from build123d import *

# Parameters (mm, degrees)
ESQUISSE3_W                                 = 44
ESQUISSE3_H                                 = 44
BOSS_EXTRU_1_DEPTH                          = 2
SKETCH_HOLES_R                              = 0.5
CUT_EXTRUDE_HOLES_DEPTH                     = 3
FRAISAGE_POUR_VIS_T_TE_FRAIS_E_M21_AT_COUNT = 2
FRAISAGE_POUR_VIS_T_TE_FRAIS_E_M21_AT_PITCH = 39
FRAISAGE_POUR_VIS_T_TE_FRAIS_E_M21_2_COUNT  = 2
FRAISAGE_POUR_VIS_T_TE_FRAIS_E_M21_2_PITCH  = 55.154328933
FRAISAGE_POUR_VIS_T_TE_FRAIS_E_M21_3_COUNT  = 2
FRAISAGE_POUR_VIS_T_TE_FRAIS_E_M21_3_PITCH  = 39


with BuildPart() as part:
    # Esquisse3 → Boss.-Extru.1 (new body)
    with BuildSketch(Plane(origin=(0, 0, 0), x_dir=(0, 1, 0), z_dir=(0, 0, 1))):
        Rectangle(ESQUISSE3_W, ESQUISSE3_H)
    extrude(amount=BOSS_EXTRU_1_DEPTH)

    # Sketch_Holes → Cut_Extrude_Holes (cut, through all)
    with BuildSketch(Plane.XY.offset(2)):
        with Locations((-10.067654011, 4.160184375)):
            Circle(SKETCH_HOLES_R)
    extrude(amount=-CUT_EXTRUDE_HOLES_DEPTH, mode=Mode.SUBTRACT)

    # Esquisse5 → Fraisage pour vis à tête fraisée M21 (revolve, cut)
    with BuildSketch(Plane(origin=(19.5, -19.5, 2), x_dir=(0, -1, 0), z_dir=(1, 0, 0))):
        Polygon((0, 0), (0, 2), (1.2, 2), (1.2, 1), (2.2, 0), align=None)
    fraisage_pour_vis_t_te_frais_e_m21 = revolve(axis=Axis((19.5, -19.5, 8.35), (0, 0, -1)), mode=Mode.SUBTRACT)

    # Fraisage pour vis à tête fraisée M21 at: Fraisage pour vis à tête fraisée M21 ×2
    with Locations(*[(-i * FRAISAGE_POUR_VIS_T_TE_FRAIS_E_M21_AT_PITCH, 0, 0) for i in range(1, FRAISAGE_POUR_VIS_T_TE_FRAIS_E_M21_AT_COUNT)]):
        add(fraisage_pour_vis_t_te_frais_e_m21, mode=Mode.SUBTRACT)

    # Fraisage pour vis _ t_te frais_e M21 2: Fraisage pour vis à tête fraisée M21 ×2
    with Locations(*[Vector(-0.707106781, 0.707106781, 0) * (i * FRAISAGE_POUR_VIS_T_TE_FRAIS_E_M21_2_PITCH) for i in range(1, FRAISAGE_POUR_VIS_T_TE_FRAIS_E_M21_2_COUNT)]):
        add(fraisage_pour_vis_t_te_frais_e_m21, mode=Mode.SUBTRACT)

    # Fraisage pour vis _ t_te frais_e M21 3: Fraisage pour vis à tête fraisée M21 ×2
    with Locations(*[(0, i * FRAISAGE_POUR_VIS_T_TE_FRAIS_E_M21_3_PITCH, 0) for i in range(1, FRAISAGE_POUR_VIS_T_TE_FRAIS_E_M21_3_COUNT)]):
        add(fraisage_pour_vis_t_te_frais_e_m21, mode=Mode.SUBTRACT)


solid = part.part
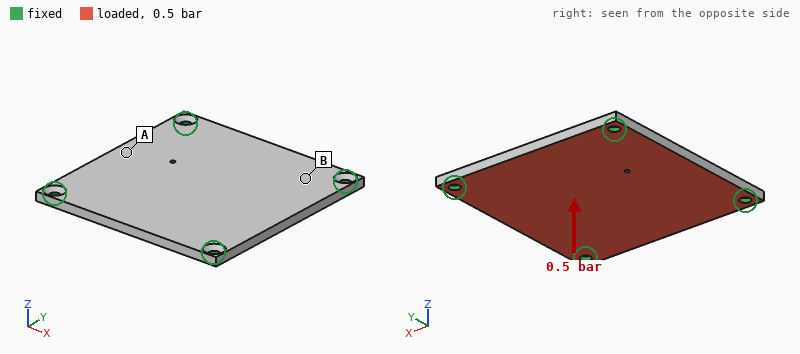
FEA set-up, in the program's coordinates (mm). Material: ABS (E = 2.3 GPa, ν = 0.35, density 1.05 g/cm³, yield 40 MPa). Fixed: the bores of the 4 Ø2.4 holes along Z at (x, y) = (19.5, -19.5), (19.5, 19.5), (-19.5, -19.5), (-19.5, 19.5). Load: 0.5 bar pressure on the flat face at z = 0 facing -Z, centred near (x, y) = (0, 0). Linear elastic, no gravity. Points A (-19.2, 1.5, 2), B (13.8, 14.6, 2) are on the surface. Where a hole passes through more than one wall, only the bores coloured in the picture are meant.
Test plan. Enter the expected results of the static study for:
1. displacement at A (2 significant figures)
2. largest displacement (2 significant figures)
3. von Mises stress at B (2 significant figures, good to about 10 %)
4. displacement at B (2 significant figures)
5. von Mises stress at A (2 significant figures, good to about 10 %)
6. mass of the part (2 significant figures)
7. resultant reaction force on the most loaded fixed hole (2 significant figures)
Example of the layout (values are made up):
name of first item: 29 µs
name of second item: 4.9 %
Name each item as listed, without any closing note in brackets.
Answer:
displacement at A: 0.39 mm
largest displacement: 0.67 mm
von Mises stress at B: 3.5 MPa
displacement at B: 0.25 mm
von Mises stress at A: 8.2 MPa
mass of the part: 4.0 g
resultant reaction force on the most loaded fixed hole: 38 N
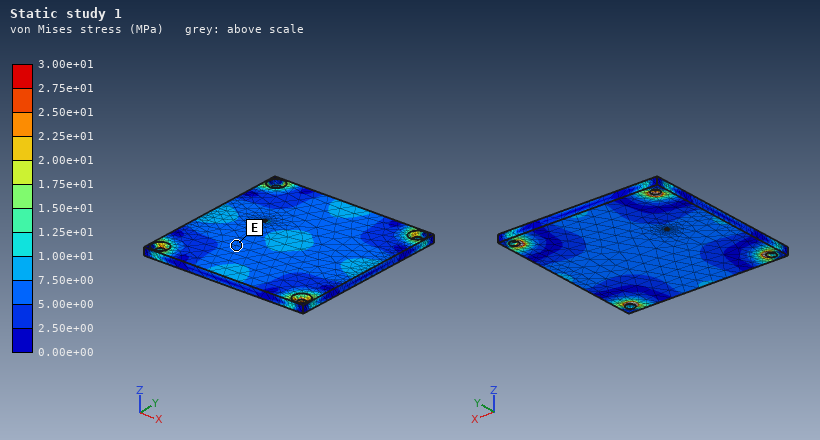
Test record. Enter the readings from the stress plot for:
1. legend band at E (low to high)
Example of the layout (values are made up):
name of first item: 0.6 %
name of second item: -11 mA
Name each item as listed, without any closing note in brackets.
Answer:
legend band at E: 5.00e+00 to 7.50e+00 MPa
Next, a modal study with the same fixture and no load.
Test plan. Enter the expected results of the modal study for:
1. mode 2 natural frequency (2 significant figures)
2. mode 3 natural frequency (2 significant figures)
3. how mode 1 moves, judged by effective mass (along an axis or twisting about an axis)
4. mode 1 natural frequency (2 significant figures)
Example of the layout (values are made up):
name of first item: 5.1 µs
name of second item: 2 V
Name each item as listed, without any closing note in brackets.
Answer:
mode 2 natural frequency: 2000 Hz
mode 3 natural frequency: 2000 Hz
how mode 1 moves, judged by effective mass: along Z
mode 1 natural frequency: 1100 Hz
